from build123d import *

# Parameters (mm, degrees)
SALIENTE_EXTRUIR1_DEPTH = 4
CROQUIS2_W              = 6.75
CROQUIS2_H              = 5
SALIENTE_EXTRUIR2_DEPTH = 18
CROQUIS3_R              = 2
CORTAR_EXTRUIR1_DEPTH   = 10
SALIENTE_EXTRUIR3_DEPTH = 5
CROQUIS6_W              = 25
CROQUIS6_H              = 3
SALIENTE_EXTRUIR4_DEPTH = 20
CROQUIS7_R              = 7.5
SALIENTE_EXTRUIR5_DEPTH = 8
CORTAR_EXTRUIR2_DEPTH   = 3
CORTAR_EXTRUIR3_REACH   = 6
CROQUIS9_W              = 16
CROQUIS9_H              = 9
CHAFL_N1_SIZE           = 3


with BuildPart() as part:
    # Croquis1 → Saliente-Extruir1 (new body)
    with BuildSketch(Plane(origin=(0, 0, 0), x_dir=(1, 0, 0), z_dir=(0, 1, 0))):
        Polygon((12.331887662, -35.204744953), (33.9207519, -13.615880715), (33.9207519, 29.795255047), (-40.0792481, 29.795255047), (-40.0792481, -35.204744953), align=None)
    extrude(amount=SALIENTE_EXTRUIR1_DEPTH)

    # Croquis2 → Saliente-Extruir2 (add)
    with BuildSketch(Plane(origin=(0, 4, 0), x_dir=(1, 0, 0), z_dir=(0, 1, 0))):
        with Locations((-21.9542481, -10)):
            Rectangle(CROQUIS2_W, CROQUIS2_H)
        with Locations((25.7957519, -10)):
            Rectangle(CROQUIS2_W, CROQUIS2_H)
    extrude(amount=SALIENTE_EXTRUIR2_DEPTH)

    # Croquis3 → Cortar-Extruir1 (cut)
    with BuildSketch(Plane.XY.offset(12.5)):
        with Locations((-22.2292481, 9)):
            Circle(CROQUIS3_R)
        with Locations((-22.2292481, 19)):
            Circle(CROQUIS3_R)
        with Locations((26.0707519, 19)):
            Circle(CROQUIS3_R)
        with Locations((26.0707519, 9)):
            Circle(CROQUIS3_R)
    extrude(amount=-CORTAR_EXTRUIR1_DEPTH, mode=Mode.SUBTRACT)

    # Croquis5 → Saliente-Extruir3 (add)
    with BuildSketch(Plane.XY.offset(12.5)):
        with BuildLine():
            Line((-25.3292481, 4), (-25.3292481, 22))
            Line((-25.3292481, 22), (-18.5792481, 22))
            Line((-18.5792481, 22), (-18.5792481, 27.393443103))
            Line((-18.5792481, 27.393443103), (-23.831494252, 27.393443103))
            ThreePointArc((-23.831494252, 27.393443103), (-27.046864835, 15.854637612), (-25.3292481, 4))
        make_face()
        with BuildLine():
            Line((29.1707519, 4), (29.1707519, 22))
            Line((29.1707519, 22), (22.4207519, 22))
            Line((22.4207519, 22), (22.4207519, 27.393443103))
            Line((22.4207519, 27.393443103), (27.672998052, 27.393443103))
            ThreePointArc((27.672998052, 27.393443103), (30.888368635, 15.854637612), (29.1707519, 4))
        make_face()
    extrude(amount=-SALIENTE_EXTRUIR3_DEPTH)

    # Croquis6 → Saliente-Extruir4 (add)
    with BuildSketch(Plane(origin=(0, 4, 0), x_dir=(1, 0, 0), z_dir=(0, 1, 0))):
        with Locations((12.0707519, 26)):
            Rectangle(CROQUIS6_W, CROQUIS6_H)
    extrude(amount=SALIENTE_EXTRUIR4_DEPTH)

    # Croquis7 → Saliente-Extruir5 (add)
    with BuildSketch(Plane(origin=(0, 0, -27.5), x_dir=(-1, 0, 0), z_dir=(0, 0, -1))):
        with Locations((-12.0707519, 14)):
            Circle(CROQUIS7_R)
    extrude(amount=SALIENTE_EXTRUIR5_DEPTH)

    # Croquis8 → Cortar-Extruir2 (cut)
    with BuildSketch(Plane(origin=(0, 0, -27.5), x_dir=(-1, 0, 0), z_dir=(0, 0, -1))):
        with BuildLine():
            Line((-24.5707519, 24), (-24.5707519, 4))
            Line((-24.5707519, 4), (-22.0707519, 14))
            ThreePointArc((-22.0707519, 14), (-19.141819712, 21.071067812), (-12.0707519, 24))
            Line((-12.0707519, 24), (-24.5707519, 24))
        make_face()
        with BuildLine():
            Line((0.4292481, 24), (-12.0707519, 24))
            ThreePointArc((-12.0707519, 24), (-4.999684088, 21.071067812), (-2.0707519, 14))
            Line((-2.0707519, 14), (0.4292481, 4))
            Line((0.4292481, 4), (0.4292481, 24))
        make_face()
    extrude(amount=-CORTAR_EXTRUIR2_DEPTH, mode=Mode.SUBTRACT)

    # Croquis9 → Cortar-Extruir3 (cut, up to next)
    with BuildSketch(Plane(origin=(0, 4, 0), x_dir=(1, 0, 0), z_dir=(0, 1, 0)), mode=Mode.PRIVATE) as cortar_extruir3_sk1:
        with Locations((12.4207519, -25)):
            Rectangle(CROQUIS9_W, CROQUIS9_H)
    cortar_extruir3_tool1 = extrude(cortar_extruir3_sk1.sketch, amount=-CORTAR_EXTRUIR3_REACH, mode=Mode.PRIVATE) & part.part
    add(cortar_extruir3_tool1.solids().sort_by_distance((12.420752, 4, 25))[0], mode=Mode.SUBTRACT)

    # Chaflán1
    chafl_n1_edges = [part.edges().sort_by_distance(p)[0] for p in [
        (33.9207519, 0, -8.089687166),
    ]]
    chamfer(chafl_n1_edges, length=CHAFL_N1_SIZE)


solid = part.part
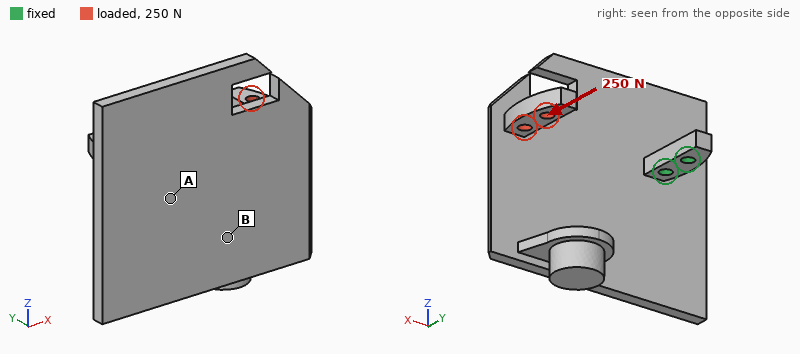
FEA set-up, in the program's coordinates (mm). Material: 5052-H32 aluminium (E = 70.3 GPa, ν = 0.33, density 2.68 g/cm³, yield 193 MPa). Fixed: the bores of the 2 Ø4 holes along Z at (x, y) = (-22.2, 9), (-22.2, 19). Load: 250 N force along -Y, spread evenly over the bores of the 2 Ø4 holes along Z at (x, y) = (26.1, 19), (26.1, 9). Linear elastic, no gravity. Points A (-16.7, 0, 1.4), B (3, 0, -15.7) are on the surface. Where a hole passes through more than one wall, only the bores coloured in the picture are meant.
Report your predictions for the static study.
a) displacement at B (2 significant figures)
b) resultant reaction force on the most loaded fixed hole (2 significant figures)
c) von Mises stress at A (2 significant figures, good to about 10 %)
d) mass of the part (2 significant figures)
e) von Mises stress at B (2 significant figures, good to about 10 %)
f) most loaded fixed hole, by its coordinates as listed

0.37 mm
440 N
75 MPa
58 g
28 MPa
(-22.2, 9)
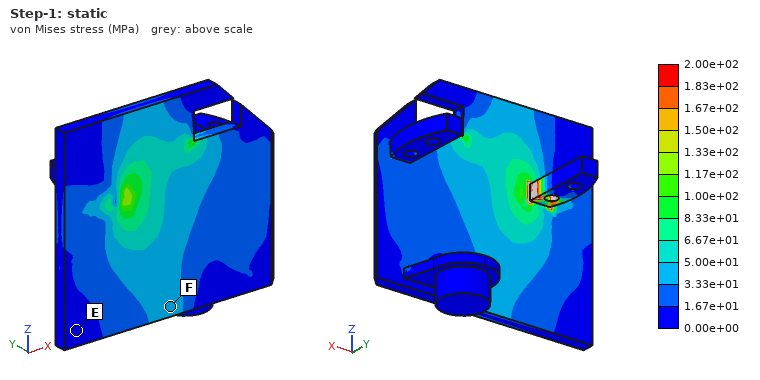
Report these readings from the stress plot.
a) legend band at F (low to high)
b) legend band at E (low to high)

3.33e+01 to 5.00e+01 MPa
0.00e+00 to 1.67e+01 MPa
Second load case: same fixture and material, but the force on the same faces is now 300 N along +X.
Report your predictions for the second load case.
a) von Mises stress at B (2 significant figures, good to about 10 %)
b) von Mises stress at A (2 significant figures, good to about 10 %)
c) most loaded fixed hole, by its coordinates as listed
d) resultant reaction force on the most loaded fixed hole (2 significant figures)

18 MPa
24 MPa
(-22.2, 9)
260 N
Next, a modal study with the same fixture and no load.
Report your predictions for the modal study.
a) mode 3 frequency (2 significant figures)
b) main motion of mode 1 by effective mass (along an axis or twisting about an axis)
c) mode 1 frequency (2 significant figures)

960 Hz
along Y
540 Hz
